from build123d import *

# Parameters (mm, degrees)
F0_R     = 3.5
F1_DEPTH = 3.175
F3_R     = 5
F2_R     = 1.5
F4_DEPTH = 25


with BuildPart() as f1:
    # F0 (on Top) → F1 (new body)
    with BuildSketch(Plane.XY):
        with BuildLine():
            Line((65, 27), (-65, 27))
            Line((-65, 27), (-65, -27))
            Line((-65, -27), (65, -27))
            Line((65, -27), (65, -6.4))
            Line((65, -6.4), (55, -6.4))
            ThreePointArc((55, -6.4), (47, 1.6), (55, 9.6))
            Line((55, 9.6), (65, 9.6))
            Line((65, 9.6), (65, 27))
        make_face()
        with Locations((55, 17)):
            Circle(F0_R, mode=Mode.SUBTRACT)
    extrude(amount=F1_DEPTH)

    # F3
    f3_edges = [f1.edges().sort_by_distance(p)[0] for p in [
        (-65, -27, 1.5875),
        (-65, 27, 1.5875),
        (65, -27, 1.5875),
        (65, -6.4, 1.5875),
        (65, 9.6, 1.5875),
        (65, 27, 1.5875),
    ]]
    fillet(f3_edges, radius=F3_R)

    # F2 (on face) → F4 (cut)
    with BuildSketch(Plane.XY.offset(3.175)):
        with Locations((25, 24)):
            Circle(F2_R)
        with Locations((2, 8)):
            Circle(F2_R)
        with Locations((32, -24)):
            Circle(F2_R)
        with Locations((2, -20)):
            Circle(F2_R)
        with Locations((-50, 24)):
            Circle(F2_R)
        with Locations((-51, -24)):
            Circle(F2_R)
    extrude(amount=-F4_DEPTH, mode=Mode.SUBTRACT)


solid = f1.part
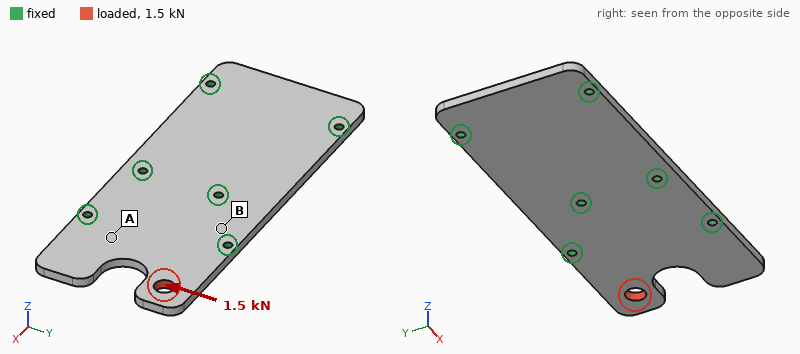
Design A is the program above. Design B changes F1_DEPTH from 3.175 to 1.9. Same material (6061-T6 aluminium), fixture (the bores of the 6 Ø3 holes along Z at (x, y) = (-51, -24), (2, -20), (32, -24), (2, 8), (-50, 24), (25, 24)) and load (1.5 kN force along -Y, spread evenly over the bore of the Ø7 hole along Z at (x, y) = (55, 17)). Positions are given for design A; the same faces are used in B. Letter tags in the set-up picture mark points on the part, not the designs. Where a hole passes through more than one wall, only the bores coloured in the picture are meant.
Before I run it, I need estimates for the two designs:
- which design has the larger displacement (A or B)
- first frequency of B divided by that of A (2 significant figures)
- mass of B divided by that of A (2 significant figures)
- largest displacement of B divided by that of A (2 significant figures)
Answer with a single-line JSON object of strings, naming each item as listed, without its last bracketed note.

{"which design has the larger displacement": "B", "first frequency of B divided by that of A": "0.62", "mass of B divided by that of A": "0.60", "largest displacement of B divided by that of A": "1.7"}
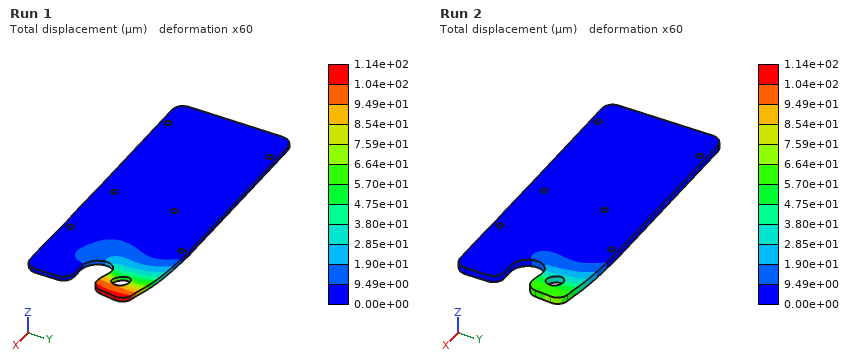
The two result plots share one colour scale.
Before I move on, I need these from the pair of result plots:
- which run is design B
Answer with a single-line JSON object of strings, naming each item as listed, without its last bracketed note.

{"which run is design B": "Run 1"}
